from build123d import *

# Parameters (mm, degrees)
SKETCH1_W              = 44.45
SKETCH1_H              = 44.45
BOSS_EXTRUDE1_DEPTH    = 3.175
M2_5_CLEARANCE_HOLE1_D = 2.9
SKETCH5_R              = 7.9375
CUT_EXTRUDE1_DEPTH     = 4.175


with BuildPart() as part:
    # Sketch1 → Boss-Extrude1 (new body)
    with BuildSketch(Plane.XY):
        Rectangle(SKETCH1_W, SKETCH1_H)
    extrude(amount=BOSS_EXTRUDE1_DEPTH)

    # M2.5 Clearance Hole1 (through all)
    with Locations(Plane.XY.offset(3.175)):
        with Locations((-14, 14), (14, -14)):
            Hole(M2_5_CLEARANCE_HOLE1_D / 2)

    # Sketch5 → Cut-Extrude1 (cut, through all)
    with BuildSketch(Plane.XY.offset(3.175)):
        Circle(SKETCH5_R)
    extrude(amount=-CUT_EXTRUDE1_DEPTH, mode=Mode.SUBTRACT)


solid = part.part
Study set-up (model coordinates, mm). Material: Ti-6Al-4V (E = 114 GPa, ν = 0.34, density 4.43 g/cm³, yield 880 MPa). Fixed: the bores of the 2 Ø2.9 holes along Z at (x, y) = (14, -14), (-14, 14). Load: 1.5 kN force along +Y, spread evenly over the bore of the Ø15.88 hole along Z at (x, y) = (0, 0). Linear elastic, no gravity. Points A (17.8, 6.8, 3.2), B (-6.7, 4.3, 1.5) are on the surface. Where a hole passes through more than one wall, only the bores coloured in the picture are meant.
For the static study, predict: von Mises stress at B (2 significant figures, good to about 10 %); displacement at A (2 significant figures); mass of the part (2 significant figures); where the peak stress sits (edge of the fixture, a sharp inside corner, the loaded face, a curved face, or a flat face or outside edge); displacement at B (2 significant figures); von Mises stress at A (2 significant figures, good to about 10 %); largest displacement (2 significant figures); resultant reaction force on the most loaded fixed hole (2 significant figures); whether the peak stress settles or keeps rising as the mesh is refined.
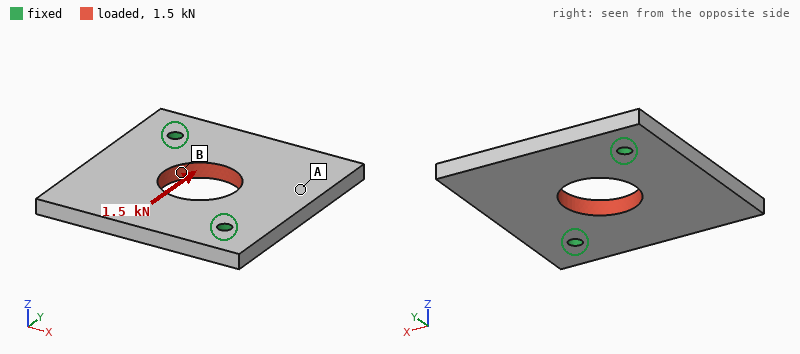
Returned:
16 MPa
1.9 µm
25 g
edge of the fixture
2.6 µm
5.6 MPa
3.5 µm
750 N
keeps rising
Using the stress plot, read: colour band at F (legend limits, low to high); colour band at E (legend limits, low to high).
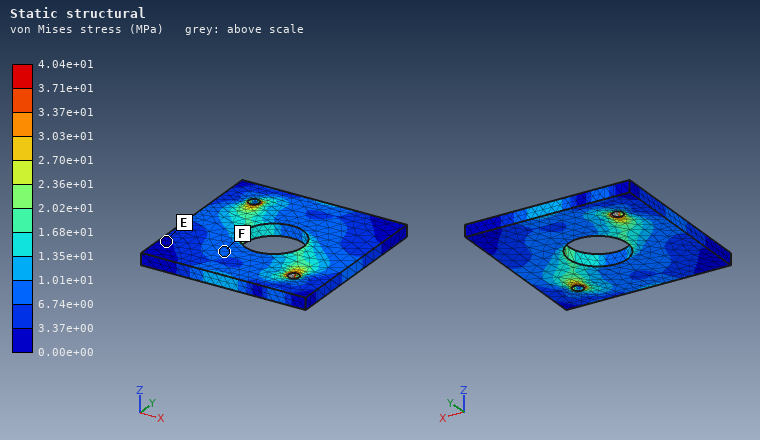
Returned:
6.74e+00 to 1.01e+01 MPa
0.00e+00 to 3.37e+00 MPa
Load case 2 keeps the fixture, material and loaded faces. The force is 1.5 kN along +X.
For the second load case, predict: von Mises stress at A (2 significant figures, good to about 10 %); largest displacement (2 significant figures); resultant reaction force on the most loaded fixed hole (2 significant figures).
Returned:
6.7 MPa
3.5 µm
750 N
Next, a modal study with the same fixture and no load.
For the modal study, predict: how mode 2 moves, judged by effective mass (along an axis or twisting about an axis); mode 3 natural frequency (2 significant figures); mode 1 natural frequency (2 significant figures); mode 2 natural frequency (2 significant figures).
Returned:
along Z
11 kHz
3200 Hz
3800 Hz
